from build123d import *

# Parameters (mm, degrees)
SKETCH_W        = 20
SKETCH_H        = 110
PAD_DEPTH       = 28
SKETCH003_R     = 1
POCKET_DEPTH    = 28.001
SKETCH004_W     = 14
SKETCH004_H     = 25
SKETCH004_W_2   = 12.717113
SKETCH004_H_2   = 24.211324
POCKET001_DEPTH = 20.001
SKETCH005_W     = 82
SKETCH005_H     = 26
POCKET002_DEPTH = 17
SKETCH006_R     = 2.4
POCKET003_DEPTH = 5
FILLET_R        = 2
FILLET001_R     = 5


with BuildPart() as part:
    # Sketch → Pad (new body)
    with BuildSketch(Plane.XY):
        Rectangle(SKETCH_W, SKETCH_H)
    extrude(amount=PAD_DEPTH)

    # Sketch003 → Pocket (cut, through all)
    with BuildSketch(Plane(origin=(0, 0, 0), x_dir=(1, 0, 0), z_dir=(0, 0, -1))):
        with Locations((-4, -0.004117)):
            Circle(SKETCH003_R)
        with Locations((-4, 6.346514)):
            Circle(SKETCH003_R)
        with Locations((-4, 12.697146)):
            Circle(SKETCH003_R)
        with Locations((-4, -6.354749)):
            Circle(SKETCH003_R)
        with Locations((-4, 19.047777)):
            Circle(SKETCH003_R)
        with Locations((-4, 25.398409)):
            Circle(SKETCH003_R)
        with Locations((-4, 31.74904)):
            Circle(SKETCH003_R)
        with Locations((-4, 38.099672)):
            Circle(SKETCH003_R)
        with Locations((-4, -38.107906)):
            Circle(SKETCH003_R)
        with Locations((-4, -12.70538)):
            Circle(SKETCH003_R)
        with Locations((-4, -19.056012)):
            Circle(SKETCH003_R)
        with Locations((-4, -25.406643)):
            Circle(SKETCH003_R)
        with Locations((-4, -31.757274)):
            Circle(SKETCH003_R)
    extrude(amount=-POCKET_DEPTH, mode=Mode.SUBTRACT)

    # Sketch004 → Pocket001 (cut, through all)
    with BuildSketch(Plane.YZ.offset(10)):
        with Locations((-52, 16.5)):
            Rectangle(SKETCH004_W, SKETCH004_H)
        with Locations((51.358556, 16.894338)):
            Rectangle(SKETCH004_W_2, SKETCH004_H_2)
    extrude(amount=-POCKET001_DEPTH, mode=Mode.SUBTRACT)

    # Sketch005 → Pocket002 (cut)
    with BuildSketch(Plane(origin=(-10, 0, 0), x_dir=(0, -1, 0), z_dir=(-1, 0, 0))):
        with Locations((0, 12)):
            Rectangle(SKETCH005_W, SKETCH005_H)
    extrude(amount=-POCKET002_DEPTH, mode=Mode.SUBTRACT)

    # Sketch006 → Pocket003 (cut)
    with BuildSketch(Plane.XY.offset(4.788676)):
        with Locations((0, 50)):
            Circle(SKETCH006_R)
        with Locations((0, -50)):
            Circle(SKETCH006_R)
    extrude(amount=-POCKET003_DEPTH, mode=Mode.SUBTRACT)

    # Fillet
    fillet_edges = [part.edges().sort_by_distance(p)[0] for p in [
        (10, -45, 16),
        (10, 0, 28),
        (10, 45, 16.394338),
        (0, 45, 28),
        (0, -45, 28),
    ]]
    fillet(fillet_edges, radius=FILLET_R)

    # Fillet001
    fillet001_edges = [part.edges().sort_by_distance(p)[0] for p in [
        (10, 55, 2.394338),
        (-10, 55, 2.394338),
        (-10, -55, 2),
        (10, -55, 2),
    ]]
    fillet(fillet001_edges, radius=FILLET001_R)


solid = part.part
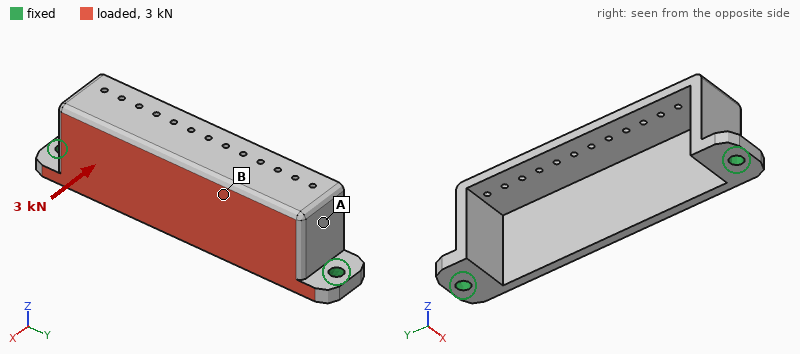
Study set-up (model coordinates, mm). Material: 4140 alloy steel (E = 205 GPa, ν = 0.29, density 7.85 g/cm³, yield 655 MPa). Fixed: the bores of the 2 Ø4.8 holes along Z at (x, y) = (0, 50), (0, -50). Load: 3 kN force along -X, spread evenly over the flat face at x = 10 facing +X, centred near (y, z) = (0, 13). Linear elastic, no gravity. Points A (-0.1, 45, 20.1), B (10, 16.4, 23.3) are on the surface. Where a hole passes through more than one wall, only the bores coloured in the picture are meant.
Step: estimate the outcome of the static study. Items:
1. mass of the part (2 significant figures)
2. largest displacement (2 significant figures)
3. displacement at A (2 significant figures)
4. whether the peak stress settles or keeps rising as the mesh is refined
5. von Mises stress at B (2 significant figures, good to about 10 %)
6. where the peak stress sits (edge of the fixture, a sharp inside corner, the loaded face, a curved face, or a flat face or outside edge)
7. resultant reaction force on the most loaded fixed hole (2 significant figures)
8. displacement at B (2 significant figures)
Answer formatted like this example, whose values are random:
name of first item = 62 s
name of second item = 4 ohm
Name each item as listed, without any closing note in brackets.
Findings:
mass of the part = 130 g
largest displacement = 0.22 mm
displacement at A = 0.034 mm
whether the peak stress settles or keeps rising as the mesh is refined = keeps rising
von Mises stress at B = 92 MPa
where the peak stress sits = edge of the fixture
resultant reaction force on the most loaded fixed hole = 1.7 kN
displacement at B = 0.087 mm
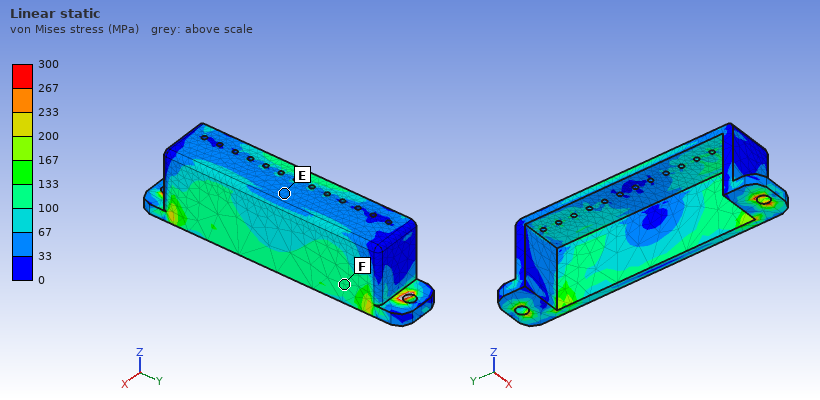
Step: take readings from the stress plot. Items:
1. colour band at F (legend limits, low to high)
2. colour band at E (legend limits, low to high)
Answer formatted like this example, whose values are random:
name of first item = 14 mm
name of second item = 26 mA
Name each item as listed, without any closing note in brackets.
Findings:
colour band at F = 100 to 133 MPa
colour band at E = 33 to 67 MPa
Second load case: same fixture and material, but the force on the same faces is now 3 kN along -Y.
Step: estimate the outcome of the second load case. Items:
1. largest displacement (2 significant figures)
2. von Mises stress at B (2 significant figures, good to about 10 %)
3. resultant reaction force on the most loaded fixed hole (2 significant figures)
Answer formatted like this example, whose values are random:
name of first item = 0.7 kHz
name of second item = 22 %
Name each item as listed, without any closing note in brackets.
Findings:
largest displacement = 13 µm
von Mises stress at B = 8.5 MPa
resultant reaction force on the most loaded fixed hole = 1.6 kN
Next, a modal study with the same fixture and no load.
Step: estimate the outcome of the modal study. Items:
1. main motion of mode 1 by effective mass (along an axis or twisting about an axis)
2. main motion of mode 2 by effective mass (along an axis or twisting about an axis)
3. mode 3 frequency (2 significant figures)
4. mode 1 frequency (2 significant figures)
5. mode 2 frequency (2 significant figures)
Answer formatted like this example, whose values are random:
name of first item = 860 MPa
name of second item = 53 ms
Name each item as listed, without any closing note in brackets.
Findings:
main motion of mode 1 by effective mass = along X
main motion of mode 2 by effective mass = twisting about Y
mode 3 frequency = 4300 Hz
mode 1 frequency = 2600 Hz
mode 2 frequency = 3300 Hz
